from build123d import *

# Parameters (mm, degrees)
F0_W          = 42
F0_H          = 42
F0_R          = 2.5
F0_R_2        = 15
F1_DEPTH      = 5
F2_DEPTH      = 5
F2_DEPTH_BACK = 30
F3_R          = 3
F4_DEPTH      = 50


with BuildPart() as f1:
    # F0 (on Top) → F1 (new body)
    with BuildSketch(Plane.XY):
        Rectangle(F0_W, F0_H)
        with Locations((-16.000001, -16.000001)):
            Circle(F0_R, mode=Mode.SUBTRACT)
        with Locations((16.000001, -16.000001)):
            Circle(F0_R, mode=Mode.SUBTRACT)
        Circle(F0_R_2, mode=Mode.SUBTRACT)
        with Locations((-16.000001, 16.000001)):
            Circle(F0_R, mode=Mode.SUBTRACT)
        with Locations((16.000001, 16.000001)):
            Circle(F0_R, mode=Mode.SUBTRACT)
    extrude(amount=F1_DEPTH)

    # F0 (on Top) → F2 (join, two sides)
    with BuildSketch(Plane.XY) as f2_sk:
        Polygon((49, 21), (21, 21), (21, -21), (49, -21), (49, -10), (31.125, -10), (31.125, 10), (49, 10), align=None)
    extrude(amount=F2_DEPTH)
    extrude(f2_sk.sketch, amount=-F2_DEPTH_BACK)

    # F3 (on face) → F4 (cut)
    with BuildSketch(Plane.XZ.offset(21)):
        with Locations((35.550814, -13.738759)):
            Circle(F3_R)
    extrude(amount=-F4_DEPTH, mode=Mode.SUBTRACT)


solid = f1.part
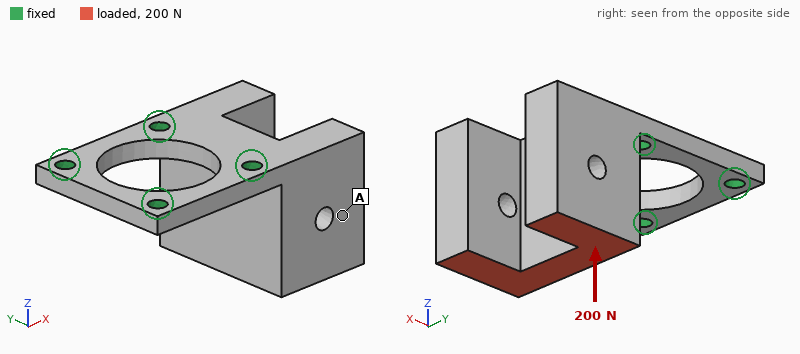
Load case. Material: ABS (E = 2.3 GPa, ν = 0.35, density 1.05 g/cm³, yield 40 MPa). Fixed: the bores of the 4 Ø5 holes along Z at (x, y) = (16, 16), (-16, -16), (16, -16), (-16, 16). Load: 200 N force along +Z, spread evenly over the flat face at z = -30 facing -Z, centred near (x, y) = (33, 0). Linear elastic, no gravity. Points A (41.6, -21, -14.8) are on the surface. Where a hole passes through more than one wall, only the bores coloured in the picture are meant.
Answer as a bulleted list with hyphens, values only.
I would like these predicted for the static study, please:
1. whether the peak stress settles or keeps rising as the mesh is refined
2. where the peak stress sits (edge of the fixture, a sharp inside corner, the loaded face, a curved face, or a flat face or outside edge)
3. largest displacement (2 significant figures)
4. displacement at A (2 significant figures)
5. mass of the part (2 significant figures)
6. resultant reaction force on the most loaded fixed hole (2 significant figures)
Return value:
- keeps rising
- edge of the fixture
- 0.95 mm
- 0.61 mm
- 35 g
- 100 N
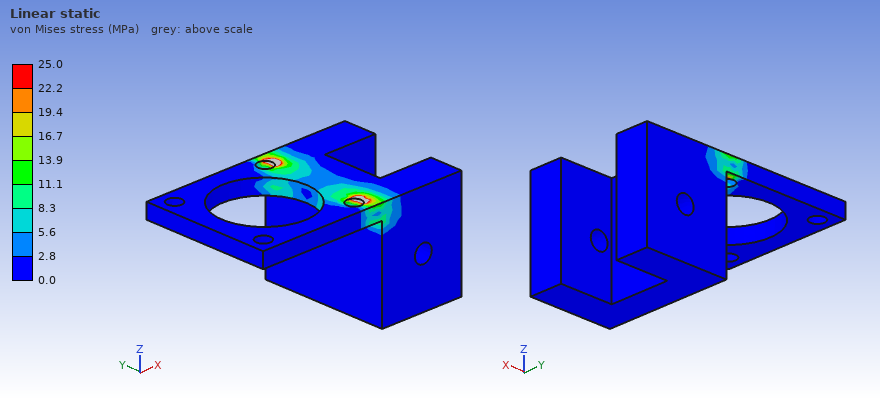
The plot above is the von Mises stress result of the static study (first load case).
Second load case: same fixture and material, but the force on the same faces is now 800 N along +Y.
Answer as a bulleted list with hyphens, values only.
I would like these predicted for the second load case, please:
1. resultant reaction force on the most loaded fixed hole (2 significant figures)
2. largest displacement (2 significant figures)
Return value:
- 960 N
- 0.66 mm
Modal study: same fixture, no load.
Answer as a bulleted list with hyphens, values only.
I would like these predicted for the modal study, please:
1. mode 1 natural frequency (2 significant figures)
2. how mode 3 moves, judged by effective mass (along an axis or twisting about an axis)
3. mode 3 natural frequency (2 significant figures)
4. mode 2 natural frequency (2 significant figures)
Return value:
- 430 Hz
- along Y
- 1800 Hz
- 1600 Hz
